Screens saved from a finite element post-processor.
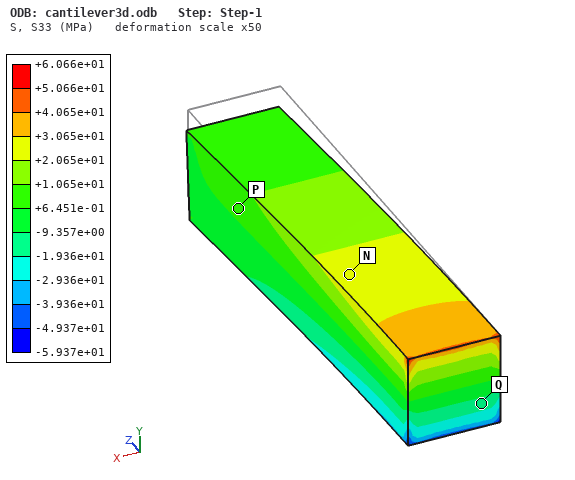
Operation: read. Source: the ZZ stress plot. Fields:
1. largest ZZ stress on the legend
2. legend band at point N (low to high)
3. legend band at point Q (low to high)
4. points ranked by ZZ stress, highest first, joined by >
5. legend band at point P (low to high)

+6.066e+01 MPa
+2.065e+01 to +3.065e+01 MPa
-1.936e+01 to -9.357e+00 MPa
N > P > Q
+6.451e-01 to +1.065e+01 MPa
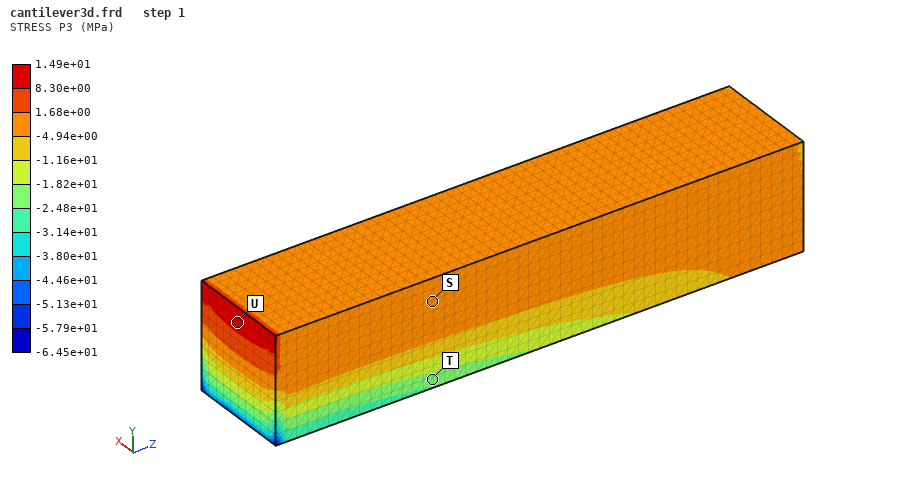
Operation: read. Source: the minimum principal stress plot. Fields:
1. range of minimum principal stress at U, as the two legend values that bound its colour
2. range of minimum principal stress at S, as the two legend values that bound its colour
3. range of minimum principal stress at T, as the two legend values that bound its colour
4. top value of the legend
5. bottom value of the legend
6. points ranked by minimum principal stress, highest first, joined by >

8.30e+00 to 1.49e+01 MPa
-4.94e+00 to 1.68e+00 MPa
-2.48e+01 to -1.82e+01 MPa
1.49e+01 MPa
-6.45e+01 MPa
U > S > T
